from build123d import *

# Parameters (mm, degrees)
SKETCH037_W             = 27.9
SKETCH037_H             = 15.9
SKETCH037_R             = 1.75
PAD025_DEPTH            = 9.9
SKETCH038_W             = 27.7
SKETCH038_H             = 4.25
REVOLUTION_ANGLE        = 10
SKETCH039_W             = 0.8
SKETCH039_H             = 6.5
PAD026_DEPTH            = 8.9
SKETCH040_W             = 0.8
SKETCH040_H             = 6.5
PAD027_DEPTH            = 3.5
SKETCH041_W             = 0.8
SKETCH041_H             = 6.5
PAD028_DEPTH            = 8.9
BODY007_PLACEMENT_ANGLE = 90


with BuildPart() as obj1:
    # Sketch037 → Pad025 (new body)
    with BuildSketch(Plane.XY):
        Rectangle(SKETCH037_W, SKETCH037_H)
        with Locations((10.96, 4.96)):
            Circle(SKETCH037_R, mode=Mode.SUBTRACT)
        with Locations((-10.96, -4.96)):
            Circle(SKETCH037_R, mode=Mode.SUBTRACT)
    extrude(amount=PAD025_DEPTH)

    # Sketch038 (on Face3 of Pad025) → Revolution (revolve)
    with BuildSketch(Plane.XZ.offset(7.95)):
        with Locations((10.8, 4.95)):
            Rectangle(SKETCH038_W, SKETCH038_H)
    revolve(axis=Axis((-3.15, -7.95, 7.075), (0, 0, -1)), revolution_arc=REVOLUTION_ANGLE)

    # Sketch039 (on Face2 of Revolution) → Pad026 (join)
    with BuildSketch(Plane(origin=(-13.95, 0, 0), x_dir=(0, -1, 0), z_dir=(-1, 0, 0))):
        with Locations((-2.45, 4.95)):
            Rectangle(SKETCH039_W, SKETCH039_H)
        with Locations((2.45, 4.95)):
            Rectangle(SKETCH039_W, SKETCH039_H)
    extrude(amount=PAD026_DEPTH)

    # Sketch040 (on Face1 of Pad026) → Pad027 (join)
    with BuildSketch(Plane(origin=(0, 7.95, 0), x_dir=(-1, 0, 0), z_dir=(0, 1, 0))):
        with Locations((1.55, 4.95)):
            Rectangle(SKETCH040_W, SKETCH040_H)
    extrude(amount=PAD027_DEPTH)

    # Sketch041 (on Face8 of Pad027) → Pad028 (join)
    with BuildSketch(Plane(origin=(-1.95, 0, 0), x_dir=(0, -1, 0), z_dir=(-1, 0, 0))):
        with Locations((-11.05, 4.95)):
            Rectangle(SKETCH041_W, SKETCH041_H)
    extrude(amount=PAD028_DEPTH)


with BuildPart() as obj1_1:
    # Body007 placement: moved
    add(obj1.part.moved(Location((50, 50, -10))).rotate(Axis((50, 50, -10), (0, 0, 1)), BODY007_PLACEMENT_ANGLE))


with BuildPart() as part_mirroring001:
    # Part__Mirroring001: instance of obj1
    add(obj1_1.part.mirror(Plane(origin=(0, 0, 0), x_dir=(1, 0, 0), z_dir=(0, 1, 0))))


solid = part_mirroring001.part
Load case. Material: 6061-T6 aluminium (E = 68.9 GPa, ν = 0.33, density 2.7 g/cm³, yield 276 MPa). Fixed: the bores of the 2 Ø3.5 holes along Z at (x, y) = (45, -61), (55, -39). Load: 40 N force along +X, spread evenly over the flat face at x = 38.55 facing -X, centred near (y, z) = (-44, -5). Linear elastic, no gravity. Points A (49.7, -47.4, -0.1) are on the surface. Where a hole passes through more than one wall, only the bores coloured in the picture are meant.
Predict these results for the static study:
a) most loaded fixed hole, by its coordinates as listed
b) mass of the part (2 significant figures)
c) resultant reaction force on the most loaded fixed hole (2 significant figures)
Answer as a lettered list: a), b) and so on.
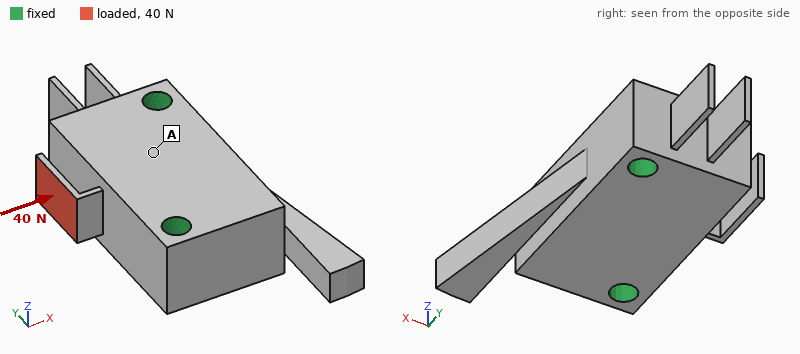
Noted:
a) (55, -39)
b) 13 g
c) 32 N
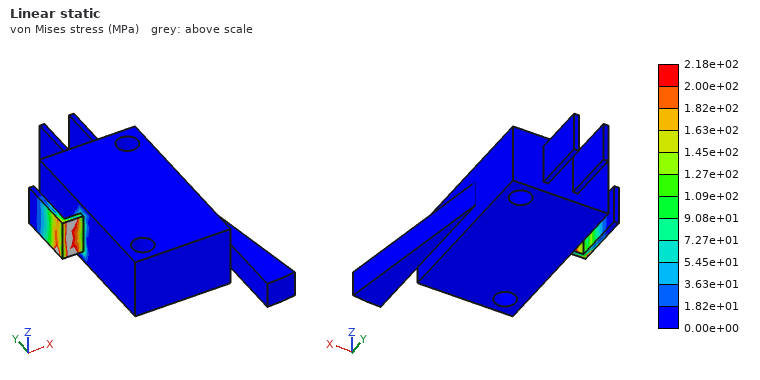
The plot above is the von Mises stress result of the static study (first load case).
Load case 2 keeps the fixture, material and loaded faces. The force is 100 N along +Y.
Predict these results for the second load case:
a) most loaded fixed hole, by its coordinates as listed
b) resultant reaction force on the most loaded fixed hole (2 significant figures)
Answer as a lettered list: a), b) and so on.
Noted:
a) (45, -61)
b) 79 N
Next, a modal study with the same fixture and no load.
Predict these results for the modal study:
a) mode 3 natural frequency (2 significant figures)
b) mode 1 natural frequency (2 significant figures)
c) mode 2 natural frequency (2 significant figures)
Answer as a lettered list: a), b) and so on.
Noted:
a) 8100 Hz
b) 5100 Hz
c) 8100 Hz
